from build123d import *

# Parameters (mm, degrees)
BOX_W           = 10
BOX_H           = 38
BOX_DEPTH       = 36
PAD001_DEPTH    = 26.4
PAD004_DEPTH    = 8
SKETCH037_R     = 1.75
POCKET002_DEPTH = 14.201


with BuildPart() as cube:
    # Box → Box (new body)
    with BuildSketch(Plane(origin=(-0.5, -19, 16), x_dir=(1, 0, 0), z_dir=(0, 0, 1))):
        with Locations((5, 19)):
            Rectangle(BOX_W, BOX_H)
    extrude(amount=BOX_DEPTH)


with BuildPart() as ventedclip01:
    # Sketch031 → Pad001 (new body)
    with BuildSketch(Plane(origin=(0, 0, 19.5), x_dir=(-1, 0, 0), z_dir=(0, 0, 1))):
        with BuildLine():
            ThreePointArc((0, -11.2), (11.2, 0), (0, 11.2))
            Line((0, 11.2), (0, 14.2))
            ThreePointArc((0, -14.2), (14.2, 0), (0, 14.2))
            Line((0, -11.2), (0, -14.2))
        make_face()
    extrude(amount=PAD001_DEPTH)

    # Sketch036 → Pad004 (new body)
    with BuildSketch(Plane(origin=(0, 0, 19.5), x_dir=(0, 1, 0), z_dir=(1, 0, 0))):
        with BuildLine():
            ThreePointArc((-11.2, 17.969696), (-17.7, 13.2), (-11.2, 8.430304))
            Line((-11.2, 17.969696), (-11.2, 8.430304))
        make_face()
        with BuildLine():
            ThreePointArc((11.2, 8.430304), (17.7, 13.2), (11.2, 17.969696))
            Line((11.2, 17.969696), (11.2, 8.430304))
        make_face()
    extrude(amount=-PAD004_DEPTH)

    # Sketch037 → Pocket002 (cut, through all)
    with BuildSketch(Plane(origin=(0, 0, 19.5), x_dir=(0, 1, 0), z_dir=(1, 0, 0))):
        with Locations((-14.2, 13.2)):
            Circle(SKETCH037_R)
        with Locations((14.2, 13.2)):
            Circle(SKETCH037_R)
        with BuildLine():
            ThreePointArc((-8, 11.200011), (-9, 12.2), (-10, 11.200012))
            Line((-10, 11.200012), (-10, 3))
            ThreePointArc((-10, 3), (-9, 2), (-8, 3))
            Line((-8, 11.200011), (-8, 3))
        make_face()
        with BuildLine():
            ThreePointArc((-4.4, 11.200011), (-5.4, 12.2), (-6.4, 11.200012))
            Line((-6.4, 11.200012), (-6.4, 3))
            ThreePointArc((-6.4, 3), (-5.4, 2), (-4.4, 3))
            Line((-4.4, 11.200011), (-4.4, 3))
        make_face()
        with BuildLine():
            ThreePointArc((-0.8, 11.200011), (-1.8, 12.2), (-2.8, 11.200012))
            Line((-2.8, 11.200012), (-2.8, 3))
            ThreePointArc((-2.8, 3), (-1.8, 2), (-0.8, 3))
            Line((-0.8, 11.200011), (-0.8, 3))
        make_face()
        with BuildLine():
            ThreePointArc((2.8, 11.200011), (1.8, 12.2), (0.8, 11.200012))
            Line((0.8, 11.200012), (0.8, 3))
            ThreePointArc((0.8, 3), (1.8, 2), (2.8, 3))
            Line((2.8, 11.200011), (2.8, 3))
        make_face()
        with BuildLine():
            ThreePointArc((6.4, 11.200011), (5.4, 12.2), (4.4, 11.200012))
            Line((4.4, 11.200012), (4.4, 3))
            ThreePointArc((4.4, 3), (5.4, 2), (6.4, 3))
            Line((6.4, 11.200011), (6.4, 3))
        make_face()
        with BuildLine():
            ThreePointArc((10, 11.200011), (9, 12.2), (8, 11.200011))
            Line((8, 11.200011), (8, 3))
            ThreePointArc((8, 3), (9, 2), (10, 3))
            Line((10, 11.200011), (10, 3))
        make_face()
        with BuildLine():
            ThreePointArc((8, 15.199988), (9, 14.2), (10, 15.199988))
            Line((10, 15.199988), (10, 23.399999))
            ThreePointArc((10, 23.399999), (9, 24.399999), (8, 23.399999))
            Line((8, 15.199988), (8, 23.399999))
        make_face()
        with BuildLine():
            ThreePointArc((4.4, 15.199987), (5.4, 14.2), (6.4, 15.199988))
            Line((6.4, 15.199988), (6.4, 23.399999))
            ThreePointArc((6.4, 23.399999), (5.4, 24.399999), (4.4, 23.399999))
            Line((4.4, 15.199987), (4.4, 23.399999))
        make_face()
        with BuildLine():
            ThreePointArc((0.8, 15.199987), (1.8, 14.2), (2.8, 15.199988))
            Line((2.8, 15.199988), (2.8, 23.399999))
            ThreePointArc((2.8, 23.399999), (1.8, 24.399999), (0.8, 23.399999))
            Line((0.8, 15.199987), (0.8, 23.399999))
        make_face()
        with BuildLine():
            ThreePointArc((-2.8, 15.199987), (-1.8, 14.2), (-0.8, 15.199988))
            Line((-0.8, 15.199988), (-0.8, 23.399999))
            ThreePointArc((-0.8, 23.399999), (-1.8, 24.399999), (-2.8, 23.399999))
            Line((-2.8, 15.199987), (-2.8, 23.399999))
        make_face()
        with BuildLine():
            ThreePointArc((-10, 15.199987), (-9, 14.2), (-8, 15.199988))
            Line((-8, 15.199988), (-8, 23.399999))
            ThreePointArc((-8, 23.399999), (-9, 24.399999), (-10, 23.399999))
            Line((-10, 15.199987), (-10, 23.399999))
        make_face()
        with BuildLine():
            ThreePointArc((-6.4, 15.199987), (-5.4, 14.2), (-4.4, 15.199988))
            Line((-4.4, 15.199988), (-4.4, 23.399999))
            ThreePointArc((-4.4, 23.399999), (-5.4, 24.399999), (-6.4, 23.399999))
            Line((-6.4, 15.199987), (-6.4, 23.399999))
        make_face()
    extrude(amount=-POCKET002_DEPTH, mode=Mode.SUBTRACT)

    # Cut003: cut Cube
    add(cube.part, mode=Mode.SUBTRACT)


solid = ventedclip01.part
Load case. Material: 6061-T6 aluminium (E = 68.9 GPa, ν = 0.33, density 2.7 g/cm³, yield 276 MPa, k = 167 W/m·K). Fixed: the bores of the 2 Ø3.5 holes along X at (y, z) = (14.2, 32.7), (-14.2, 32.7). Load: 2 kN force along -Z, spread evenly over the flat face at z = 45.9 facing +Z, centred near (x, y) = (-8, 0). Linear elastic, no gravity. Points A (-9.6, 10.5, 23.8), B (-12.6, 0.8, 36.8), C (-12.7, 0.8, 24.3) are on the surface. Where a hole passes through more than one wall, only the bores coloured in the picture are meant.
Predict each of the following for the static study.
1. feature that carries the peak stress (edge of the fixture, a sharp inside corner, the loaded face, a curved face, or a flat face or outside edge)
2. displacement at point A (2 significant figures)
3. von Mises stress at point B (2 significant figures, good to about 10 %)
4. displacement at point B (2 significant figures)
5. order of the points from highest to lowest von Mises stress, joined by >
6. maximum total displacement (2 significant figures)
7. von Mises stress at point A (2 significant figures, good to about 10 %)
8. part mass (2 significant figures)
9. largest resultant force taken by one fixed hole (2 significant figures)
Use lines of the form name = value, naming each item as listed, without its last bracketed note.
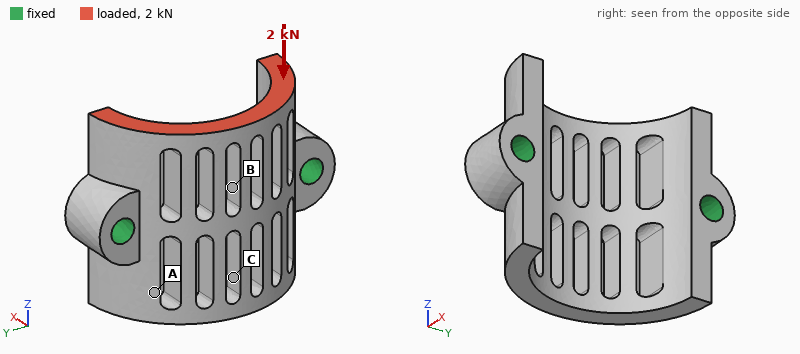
feature that carries the peak stress = a curved face
displacement at point A = 11 µm
von Mises stress at point B = 28 MPa
displacement at point B = 47 µm
order of the points from highest to lowest von Mises stress, joined by > = A > B > C
maximum total displacement = 63 µm
von Mises stress at point A = 47 MPa
part mass = 7.0 g
largest resultant force taken by one fixed hole = 1.0 kN
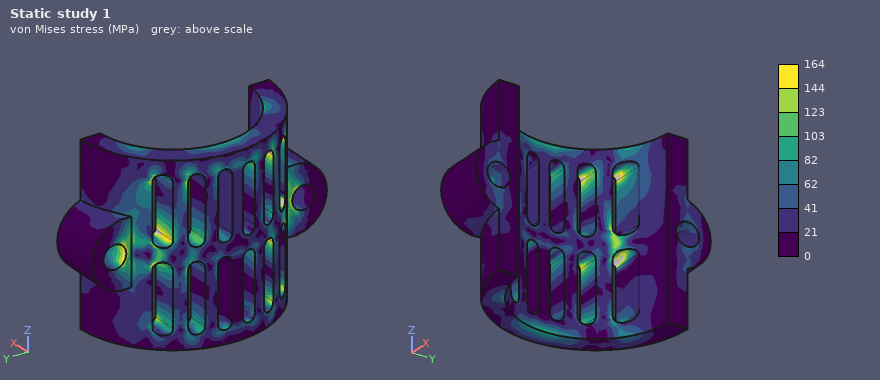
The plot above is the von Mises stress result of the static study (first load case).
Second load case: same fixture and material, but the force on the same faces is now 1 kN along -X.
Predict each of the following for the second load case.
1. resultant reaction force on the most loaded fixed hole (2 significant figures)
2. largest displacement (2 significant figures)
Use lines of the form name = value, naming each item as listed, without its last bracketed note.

resultant reaction force on the most loaded fixed hole = 550 N
largest displacement = 68 µm
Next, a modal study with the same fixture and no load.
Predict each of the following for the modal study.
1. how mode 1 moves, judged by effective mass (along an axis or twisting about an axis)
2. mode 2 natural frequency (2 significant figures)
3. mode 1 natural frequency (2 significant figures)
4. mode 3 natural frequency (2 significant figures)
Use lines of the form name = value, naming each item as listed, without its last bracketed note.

how mode 1 moves, judged by effective mass = along Z
mode 2 natural frequency = 17 kHz
mode 1 natural frequency = 15 kHz
mode 3 natural frequency = 17 kHz
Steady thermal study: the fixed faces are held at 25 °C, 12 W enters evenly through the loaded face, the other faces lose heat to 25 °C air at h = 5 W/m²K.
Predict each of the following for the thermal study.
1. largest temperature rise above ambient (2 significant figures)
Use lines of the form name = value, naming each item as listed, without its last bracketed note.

largest temperature rise above ambient = 19 K
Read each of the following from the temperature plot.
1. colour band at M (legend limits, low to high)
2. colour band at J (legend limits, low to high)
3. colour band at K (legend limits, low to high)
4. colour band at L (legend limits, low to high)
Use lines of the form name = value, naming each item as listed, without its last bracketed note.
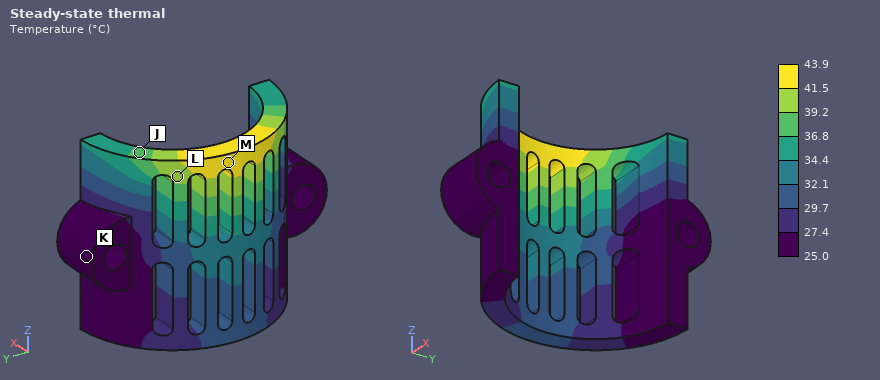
colour band at M = 41.5 to 43.9 °C
colour band at J = 36.8 to 39.2 °C
colour band at K = 25.0 to 27.4 °C
colour band at L = 39.2 to 41.5 °C
